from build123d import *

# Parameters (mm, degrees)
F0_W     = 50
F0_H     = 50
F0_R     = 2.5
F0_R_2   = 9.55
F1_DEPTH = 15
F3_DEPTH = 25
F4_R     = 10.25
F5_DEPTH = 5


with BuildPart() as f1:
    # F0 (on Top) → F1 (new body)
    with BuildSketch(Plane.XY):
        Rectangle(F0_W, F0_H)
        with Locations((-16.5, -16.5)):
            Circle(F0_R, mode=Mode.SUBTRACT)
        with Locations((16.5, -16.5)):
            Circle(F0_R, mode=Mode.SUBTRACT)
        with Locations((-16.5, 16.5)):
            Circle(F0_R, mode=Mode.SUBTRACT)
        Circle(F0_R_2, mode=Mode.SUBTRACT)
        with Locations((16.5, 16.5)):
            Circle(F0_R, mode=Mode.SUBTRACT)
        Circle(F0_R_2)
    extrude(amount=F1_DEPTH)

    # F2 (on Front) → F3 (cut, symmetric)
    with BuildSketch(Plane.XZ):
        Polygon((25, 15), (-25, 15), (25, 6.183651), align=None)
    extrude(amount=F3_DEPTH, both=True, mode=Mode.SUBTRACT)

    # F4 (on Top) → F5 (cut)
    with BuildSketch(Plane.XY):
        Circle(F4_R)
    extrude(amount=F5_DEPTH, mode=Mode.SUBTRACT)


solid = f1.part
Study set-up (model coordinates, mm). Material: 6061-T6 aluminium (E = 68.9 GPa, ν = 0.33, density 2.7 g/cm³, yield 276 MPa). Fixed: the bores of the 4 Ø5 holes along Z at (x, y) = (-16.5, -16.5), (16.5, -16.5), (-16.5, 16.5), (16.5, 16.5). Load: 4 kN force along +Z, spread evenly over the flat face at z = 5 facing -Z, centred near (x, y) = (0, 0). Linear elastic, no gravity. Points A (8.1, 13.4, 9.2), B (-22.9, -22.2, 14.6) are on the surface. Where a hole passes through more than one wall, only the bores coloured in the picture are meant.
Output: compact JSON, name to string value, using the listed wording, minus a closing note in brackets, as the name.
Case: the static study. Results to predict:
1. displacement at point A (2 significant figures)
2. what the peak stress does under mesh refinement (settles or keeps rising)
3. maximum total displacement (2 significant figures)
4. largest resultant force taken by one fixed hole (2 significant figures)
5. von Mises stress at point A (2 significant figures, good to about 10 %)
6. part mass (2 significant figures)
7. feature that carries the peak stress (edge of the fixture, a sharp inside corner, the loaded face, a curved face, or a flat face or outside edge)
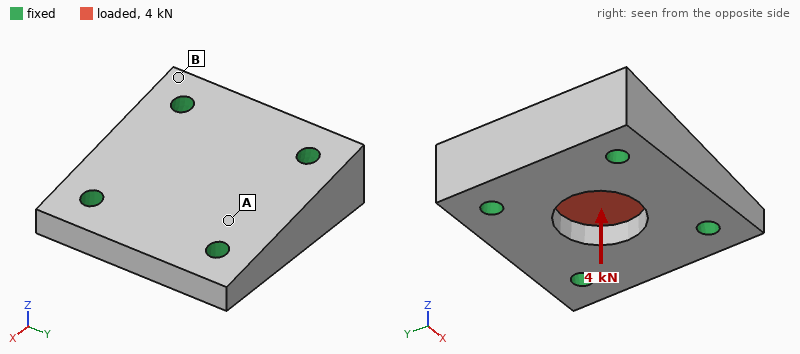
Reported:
{"displacement at point A": "5.1 µm", "what the peak stress does under mesh refinement": "keeps rising", "maximum total displacement": "17 µm", "largest resultant force taken by one fixed hole": "1.2 kN", "von Mises stress at point A": "13 MPa", "part mass": "65 g", "feature that carries the peak stress": "edge of the fixture"}
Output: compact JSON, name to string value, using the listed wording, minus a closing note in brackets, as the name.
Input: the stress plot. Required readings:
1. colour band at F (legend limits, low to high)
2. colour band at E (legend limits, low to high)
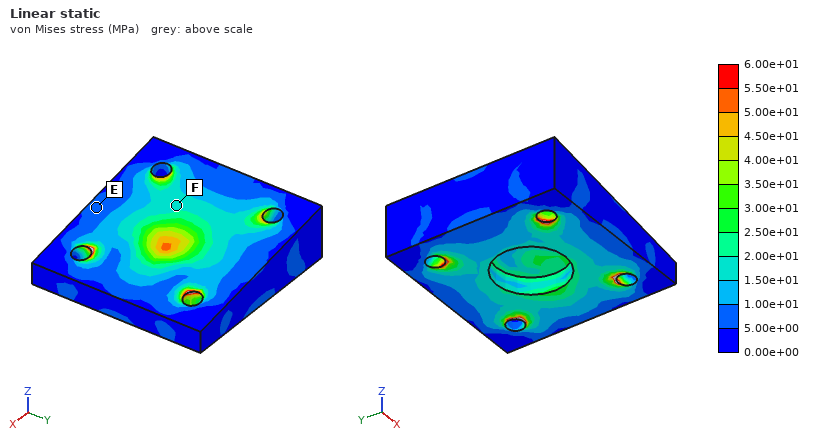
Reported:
{"colour band at F": "1.50e+01 to 2.00e+01 MPa", "colour band at E": "5.00e+00 to 1.00e+01 MPa"}
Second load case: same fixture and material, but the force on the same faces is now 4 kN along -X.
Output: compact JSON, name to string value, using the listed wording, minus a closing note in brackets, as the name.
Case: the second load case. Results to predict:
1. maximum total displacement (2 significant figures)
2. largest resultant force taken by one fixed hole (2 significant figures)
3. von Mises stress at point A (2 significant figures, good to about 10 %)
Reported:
{"maximum total displacement": "6.2 µm", "largest resultant force taken by one fixed hole": "1.3 kN", "von Mises stress at point A": "8.4 MPa"}
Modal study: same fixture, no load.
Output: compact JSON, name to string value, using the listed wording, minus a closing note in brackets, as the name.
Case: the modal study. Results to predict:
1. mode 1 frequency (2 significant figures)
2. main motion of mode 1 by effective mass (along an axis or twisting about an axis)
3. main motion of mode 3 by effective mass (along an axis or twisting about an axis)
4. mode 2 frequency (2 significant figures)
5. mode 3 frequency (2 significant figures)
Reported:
{"mode 1 frequency": "27 kHz", "main motion of mode 1 by effective mass": "along Z", "main motion of mode 3 by effective mass": "twisting about X", "mode 2 frequency": "32 kHz", "mode 3 frequency": "34 kHz"}
